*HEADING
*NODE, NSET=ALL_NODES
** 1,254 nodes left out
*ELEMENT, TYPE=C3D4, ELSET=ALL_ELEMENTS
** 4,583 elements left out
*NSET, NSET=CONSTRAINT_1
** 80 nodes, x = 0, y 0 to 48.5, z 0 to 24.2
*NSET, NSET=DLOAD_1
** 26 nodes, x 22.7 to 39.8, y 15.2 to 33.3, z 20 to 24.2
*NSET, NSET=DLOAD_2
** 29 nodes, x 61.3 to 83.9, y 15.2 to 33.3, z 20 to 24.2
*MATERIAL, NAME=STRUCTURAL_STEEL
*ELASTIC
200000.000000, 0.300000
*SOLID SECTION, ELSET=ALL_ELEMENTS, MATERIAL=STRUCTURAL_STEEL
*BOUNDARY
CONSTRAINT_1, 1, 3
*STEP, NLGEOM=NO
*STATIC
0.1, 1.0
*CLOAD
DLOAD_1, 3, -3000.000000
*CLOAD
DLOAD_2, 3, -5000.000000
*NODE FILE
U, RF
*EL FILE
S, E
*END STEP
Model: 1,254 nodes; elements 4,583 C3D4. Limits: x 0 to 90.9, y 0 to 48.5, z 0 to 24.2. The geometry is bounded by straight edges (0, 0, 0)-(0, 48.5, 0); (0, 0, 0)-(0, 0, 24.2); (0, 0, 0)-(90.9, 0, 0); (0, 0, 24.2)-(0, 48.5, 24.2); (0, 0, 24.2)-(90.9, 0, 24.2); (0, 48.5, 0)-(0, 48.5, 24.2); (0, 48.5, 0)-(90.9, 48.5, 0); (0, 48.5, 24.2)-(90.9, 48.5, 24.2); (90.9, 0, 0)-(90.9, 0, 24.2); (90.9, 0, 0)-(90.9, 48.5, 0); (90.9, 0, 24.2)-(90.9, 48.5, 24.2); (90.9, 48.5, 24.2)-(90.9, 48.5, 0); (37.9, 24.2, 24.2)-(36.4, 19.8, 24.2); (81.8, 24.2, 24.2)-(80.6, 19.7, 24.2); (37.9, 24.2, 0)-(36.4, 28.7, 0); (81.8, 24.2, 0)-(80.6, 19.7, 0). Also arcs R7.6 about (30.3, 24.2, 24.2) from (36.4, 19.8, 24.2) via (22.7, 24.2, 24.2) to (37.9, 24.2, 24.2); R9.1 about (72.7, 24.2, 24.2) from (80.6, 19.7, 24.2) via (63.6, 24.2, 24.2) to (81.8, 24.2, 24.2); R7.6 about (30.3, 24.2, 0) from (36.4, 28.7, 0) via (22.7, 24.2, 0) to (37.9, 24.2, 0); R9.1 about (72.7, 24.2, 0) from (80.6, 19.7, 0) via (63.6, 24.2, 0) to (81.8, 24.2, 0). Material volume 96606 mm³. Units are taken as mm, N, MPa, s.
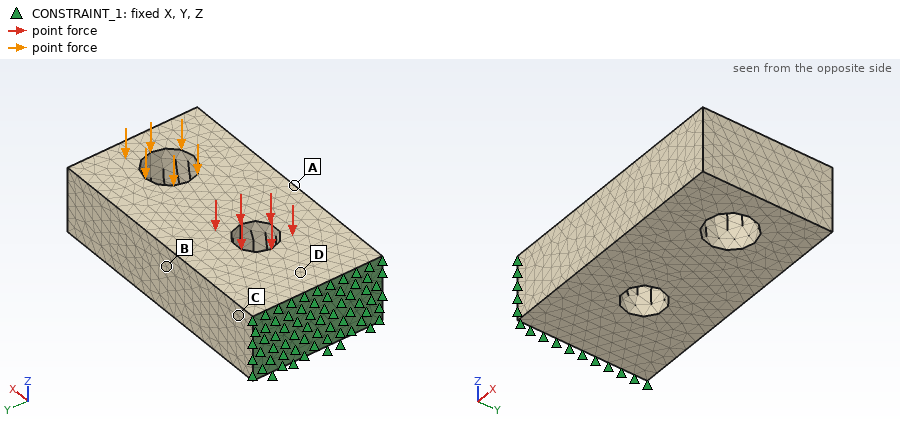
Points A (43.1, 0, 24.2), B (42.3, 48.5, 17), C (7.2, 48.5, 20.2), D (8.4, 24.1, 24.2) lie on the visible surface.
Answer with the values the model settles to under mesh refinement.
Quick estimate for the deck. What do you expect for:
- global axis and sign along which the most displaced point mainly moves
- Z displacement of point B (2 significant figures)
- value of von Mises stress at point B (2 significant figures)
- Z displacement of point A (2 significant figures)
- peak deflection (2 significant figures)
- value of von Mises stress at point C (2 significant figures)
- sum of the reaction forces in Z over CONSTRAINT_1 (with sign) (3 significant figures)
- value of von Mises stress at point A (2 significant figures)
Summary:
-Z
-0.89 mm
730 MPa
-0.92 mm
3.0 mm
1500 MPa
2.23e+05 N
1100 MPa
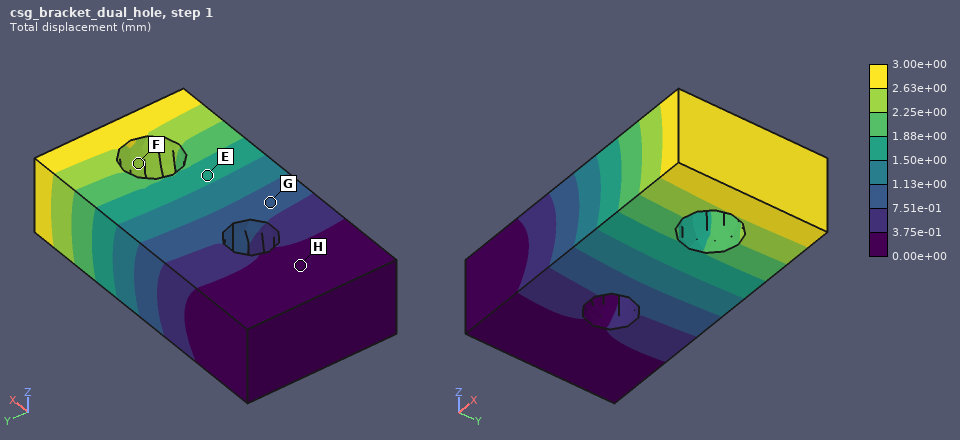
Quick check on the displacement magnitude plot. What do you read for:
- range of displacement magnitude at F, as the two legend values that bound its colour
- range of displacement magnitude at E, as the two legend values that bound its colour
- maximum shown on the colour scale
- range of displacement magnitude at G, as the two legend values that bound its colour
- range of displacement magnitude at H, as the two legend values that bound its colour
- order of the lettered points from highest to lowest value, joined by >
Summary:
2.25e+00 to 2.63e+00 mm
1.50e+00 to 1.88e+00 mm
3.00e+00 mm
7.51e-01 to 1.13e+00 mm
0.00e+00 to 3.75e-01 mm
F > E > G > H
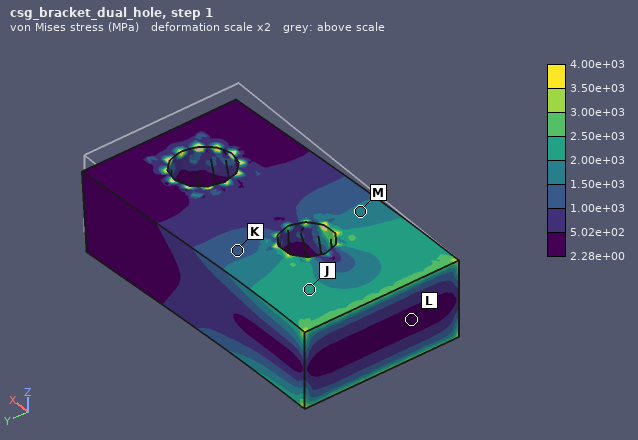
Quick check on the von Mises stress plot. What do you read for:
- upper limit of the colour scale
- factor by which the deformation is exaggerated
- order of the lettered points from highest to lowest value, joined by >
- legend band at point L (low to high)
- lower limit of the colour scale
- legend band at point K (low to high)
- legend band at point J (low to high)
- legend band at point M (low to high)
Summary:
4.00e+03 MPa
2
J > M > K > L
2.28e+00 to 5.02e+02 MPa
2.28e+00 MPa
1.00e+03 to 1.50e+03 MPa
2.00e+03 to 2.50e+03 MPa
1.50e+03 to 2.00e+03 MPa
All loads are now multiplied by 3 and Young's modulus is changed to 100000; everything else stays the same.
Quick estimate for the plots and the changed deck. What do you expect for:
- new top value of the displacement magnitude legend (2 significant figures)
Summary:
18 mm
